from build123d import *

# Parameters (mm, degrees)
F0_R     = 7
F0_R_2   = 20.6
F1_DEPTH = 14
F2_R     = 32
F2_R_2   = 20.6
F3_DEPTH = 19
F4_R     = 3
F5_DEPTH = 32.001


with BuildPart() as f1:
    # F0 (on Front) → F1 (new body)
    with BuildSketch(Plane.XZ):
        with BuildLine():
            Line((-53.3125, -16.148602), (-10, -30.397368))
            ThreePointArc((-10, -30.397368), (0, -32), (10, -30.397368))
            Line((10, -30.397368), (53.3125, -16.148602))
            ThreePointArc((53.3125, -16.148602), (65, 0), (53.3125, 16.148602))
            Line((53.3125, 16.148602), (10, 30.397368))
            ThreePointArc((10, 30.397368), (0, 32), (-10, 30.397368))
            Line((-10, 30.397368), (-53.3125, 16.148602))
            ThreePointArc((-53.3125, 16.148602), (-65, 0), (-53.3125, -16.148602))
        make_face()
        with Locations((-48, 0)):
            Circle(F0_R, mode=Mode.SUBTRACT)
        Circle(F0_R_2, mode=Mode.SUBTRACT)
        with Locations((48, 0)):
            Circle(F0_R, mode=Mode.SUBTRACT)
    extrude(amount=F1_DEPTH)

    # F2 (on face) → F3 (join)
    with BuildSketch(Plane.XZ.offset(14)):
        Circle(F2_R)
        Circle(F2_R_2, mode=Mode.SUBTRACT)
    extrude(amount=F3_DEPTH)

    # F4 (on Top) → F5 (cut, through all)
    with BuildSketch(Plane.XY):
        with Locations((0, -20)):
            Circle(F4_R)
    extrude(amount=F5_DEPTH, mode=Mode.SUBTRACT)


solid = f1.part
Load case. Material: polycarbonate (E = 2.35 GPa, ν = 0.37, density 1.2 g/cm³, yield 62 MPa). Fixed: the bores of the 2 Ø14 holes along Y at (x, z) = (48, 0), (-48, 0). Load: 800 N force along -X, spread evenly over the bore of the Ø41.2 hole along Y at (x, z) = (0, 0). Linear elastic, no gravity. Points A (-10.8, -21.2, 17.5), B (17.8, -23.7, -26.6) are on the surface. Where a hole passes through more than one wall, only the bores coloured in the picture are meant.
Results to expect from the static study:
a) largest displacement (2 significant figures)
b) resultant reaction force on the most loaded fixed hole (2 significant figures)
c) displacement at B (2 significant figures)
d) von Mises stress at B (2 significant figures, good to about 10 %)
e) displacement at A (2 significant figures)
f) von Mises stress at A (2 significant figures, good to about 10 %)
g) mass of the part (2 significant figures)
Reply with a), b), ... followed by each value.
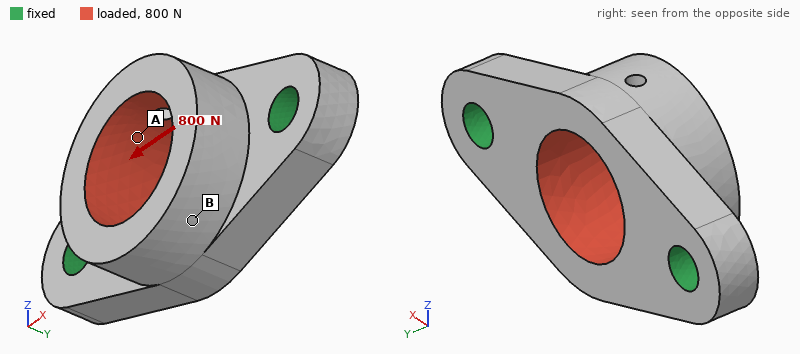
a) 21 µm
b) 410 N
c) 17 µm
d) 0.27 MPa
e) 16 µm
f) 0.74 MPa
g) 110 g
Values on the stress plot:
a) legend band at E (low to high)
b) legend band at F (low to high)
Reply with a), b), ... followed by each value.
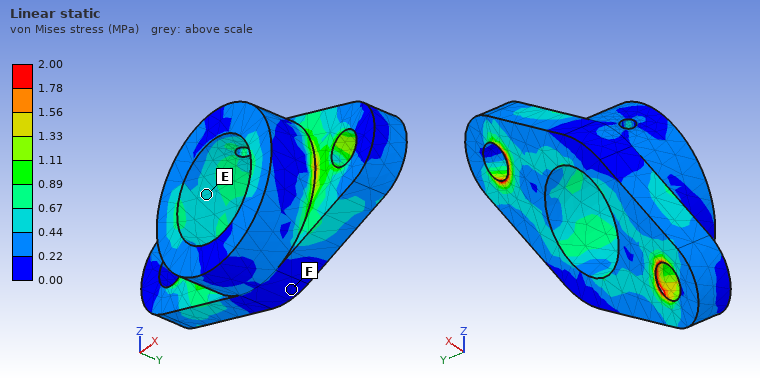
a) 0.44 to 0.67 MPa
b) 0.00 to 0.22 MPa
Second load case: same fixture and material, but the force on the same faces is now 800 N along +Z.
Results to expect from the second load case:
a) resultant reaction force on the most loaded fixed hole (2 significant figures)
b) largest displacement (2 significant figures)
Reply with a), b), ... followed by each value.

a) 400 N
b) 0.12 mm
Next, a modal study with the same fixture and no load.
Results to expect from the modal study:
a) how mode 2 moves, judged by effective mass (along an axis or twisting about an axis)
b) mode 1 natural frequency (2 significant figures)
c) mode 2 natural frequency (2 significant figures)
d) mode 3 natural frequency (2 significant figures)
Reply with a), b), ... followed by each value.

a) along Y
b) 1400 Hz
c) 2000 Hz
d) 3300 Hz
